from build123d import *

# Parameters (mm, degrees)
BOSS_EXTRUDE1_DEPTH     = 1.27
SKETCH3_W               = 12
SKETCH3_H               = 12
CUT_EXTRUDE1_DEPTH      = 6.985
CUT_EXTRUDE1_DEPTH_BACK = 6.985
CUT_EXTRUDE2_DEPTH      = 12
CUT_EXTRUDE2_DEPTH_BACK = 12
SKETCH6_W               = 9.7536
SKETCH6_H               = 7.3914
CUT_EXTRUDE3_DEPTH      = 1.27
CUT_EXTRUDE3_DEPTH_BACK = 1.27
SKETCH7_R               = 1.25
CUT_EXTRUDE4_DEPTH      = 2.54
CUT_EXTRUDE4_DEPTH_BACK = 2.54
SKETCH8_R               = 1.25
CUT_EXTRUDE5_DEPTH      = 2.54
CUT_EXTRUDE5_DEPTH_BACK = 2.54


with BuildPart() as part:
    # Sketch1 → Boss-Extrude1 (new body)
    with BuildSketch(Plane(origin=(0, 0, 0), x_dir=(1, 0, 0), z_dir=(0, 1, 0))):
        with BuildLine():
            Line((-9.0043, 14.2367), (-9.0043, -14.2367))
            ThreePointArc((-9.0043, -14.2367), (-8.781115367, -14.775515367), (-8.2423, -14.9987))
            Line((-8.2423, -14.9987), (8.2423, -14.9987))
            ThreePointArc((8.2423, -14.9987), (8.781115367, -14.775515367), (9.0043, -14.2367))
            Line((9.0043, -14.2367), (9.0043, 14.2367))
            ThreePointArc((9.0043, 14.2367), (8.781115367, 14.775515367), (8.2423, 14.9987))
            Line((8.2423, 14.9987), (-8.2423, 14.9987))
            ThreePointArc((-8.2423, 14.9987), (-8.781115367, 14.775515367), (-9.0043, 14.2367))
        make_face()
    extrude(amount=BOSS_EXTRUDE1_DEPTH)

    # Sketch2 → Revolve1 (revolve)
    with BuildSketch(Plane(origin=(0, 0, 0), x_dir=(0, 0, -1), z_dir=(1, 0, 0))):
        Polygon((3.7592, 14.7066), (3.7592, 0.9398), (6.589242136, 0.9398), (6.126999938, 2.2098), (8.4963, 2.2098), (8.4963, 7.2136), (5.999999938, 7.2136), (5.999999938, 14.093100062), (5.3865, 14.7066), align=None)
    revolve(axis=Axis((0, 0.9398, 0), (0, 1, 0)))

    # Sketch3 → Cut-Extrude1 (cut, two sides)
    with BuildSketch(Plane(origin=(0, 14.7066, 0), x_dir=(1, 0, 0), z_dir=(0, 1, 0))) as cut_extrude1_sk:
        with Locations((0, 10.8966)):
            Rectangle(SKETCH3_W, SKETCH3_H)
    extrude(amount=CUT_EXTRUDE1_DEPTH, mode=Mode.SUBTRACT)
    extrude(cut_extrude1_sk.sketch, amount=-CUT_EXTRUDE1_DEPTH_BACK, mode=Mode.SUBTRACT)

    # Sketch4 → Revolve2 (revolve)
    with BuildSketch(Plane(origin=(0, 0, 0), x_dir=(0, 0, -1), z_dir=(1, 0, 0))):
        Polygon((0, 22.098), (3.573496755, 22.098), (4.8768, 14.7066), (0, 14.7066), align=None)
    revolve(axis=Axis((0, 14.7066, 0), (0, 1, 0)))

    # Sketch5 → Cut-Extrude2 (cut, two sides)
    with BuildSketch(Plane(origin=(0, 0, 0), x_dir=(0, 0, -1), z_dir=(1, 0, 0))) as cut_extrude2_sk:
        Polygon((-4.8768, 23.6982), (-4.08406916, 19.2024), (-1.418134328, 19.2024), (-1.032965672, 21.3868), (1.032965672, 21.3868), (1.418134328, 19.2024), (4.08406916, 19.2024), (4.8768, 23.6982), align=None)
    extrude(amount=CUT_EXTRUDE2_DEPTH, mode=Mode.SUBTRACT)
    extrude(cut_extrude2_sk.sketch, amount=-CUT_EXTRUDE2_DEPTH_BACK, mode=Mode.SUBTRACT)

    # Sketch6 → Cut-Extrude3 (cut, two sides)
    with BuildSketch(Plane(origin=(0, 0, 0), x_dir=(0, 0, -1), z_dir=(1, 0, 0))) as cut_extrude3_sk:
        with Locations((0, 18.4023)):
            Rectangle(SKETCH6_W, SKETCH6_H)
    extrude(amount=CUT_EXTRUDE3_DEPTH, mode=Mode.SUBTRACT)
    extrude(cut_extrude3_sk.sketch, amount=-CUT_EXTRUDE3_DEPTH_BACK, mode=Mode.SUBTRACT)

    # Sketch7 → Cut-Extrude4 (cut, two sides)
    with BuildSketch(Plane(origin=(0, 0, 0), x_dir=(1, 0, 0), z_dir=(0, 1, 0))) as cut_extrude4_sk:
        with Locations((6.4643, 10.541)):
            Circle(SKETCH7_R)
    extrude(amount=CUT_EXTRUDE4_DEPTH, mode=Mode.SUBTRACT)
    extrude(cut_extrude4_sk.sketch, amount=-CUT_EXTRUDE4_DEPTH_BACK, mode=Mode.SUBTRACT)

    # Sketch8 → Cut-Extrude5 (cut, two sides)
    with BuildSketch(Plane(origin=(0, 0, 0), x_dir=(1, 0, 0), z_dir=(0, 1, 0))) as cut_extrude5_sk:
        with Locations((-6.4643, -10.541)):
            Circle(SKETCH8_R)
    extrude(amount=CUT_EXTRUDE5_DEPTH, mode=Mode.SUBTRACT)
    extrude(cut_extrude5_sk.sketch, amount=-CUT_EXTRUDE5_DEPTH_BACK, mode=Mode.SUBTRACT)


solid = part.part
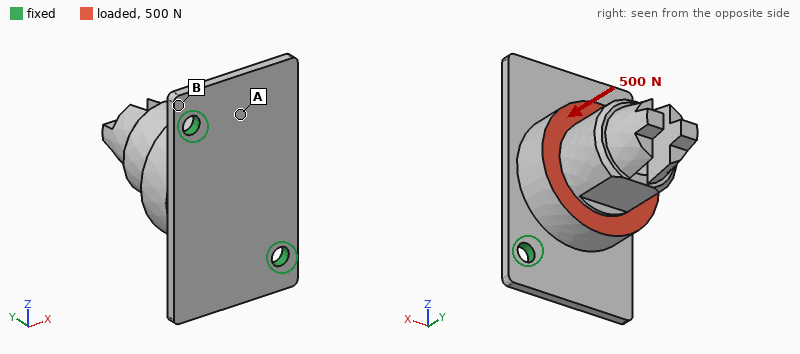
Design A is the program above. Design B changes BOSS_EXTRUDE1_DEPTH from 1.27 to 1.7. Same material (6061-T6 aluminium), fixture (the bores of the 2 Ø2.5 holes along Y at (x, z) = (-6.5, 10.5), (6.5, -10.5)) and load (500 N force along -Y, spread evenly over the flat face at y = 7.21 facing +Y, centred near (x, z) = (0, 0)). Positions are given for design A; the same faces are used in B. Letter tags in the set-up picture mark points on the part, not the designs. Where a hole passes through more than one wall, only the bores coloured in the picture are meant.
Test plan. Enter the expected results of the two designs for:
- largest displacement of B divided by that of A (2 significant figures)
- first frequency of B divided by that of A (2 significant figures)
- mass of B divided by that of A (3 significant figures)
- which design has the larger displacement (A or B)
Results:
0.56
1.4
1.08
A
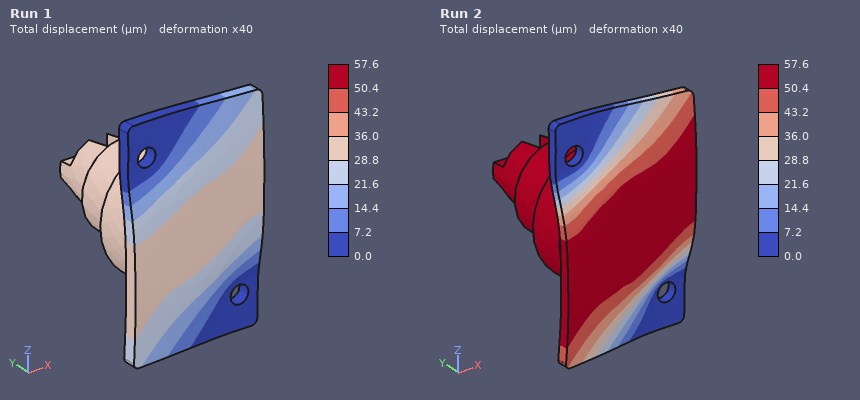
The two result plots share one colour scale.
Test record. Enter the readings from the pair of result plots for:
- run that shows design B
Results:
Run 1
